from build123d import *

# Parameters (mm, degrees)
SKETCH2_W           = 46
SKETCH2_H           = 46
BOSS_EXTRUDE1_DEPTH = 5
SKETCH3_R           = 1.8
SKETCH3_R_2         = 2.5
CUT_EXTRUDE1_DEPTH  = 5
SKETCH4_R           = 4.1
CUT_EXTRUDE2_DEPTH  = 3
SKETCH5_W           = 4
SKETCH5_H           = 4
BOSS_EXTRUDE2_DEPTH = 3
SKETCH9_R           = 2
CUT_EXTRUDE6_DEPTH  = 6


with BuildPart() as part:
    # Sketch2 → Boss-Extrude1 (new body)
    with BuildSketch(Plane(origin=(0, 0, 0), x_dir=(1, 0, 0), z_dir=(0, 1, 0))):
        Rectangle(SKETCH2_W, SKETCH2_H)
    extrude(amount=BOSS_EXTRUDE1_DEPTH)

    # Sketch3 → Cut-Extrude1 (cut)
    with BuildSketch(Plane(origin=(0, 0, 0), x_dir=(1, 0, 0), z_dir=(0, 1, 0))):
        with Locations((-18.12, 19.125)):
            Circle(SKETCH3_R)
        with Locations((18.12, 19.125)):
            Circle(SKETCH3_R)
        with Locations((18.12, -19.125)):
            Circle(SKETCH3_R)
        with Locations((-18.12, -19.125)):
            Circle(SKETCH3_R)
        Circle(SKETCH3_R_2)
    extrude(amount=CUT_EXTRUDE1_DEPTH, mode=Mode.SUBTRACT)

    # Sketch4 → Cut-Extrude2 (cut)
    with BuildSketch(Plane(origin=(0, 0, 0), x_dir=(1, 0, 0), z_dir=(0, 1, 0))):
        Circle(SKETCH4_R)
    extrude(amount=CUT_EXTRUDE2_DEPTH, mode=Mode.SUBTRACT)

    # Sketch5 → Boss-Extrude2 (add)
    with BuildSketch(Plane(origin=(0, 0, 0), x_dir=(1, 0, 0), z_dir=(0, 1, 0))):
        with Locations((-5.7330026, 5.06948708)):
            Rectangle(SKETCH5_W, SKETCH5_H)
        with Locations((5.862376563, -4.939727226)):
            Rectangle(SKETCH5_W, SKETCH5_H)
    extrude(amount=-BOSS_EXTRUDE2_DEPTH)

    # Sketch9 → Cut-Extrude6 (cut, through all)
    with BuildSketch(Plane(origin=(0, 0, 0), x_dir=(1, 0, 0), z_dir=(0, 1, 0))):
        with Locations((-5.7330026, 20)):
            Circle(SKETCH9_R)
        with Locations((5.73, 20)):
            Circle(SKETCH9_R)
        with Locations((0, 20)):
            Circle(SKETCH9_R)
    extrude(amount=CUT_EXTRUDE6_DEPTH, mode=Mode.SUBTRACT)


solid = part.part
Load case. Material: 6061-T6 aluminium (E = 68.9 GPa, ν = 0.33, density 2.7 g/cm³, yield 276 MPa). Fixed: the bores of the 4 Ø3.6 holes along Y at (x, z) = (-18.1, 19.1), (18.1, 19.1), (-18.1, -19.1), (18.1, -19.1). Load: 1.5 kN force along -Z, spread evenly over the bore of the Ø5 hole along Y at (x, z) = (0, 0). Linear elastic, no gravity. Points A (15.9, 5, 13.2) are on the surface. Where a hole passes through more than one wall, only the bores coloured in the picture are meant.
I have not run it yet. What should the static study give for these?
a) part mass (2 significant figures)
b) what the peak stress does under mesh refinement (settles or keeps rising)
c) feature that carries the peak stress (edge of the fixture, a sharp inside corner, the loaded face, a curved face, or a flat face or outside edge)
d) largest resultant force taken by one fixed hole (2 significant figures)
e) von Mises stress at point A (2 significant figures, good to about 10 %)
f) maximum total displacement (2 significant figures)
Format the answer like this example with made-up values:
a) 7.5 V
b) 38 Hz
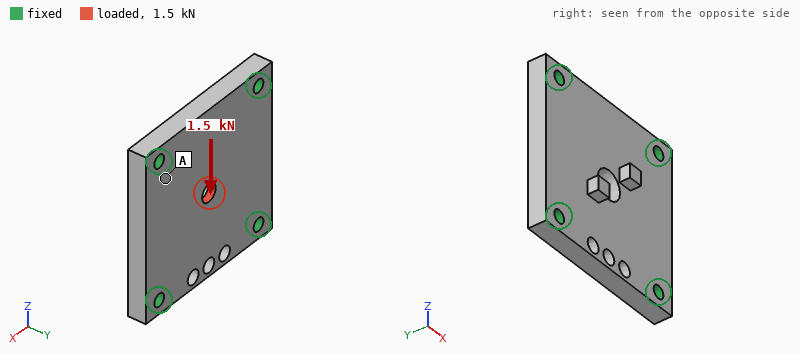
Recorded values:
a) 27 g
b) keeps rising
c) a sharp inside corner
d) 430 N
e) 8.6 MPa
f) 6.2 µm
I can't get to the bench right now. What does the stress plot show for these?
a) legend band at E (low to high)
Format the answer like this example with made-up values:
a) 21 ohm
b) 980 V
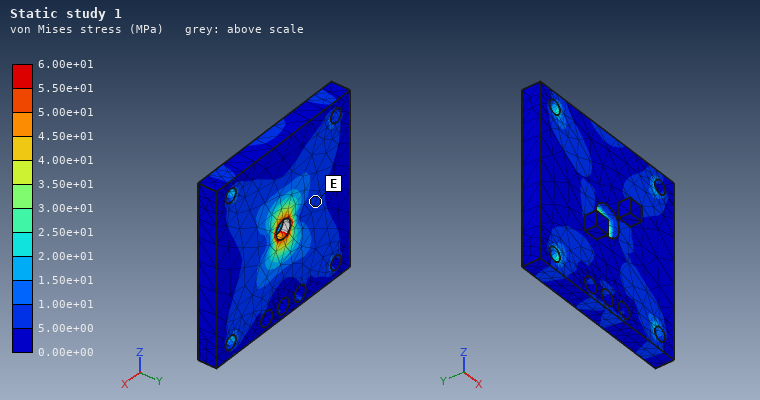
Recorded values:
a) 5.00e+00 to 1.00e+01 MPa
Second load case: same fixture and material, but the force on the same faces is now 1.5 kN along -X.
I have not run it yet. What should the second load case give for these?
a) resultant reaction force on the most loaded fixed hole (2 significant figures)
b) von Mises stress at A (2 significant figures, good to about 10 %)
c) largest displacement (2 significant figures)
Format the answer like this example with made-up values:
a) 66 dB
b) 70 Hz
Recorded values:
a) 430 N
b) 7.8 MPa
c) 6.3 µm
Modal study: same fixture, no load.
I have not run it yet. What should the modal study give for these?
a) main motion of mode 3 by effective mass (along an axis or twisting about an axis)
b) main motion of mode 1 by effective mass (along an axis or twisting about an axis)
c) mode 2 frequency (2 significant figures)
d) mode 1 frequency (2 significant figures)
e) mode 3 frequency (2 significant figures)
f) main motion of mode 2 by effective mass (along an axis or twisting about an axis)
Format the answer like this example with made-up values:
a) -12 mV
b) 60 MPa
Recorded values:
a) twisting about X
b) along Y
c) 18 kHz
d) 12 kHz
e) 20 kHz
f) twisting about Z
